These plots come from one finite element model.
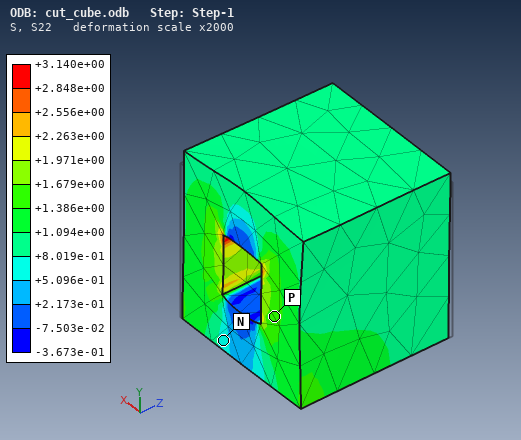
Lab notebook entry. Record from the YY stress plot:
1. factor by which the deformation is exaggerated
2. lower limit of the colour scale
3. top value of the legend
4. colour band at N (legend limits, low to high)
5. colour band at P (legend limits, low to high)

2000
-3.673e-01
+3.140e+00
+5.096e-01 to +8.019e-01
+1.386e+00 to +1.679e+00
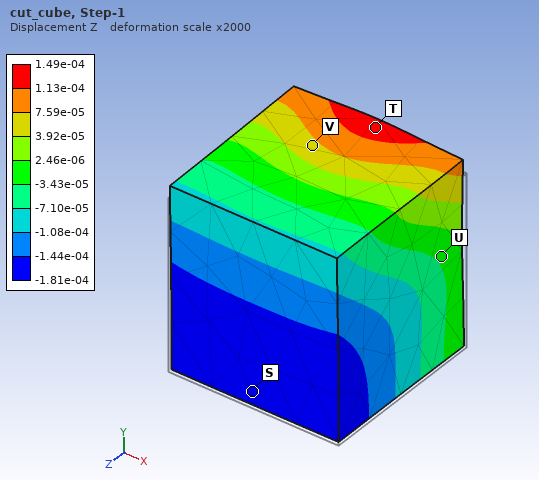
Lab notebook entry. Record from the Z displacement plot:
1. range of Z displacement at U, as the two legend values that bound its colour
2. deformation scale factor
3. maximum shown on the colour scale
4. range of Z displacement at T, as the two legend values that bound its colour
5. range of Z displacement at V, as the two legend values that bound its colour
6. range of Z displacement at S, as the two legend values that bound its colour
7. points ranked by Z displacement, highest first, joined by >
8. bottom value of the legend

-3.43e-05 to 2.46e-06
2000
1.49e-04
1.13e-04 to 1.49e-04
3.92e-05 to 7.59e-05
-1.81e-04 to -1.44e-04
T > V > U > S
-1.81e-04
